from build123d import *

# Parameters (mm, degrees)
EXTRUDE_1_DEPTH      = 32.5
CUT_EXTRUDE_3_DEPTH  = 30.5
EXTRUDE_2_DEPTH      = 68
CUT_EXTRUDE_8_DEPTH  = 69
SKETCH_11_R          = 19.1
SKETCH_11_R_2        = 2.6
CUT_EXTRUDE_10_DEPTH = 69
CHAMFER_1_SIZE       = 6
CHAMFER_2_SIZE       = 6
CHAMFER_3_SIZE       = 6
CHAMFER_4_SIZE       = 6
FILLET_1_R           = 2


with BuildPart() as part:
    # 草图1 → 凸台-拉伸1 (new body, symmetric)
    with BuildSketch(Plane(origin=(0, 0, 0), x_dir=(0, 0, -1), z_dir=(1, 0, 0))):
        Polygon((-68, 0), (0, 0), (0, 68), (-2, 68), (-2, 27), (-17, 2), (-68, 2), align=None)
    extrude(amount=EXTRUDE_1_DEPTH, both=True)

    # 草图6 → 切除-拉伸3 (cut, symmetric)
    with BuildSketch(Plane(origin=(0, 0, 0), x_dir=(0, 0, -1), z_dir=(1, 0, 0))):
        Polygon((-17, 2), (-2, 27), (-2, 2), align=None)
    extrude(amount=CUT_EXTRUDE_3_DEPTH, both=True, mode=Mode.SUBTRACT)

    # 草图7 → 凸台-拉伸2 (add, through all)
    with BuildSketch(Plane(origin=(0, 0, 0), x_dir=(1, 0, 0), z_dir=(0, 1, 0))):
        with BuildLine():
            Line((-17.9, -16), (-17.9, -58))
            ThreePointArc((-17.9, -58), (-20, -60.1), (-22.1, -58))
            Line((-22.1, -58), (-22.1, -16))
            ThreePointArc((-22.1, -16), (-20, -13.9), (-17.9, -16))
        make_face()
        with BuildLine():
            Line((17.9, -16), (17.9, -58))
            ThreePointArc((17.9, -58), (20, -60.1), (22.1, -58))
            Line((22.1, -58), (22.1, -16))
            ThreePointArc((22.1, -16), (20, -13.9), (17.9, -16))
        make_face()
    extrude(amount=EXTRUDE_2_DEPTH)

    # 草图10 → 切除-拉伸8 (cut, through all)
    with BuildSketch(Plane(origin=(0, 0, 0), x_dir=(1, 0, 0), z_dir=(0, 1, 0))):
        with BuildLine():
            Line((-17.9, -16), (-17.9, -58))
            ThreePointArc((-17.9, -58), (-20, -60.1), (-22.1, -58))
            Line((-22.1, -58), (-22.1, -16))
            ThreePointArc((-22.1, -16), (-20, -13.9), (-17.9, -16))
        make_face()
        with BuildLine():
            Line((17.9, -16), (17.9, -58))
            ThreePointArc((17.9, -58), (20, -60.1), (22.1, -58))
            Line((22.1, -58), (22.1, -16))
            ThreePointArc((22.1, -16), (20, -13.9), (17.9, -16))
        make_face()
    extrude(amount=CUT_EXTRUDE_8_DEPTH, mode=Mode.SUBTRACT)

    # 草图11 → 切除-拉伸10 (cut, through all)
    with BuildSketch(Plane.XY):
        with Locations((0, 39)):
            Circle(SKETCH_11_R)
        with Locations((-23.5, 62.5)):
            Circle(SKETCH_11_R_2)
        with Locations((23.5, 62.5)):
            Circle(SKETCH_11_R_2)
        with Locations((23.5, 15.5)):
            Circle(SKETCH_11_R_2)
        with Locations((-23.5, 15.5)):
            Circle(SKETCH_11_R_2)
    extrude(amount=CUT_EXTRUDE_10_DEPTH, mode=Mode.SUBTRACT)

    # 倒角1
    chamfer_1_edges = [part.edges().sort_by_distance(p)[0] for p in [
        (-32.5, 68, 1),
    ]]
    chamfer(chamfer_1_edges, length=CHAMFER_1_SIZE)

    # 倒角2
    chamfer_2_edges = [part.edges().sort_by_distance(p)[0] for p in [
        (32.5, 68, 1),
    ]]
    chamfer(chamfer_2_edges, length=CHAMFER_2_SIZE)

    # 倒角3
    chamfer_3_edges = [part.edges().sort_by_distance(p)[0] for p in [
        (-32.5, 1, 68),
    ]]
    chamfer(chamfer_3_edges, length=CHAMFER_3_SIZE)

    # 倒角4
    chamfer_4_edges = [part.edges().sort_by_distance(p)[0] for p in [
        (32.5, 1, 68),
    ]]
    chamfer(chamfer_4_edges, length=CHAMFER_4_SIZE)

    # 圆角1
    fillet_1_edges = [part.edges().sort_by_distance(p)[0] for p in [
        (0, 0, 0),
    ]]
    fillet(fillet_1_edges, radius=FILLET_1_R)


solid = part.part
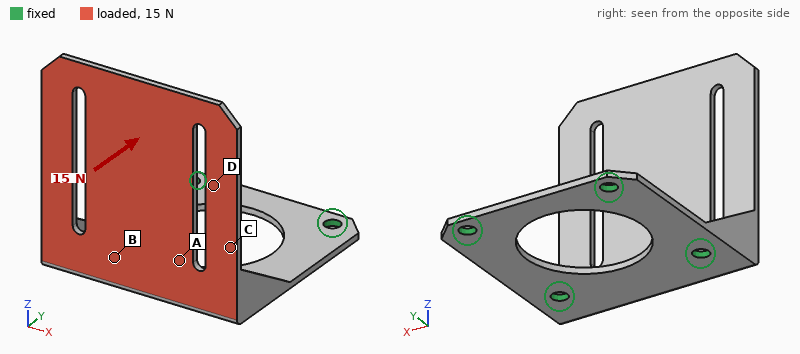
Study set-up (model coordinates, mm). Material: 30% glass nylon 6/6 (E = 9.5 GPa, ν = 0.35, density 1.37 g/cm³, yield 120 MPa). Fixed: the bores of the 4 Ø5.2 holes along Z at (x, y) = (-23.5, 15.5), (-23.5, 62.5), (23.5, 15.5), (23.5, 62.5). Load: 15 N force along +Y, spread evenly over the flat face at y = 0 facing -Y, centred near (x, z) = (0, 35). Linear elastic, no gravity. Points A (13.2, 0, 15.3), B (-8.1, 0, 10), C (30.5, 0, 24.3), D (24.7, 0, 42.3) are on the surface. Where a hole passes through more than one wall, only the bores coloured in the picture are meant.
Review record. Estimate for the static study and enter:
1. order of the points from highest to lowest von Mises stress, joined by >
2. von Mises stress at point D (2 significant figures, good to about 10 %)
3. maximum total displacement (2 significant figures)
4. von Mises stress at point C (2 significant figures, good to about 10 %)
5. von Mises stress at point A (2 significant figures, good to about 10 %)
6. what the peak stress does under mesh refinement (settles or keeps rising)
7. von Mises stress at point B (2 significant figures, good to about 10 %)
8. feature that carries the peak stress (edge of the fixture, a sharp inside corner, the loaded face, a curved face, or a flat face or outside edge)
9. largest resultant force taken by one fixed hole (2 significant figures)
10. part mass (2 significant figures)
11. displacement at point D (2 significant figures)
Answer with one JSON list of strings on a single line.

["C > A > B > D", "2.9 MPa", "1.4 mm", "8.6 MPa", "6.6 MPa", "keeps rising", "5.1 MPa", "a sharp inside corner", "9.1 N", "20 g", "0.60 mm"]
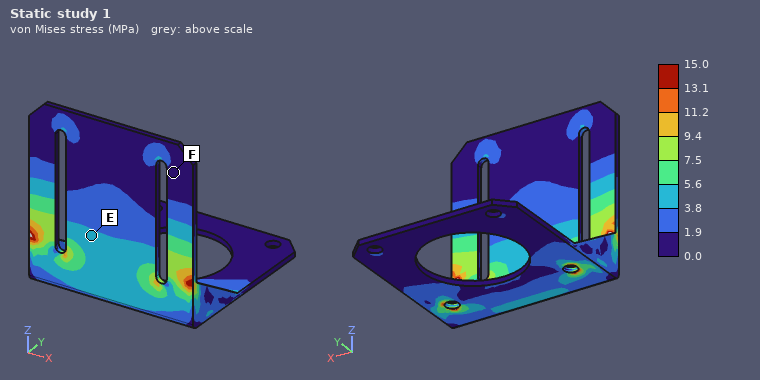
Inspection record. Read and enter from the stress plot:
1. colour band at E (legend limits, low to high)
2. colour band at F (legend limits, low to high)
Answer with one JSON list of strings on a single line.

["3.8 to 5.6 MPa", "0.0 to 1.9 MPa"]
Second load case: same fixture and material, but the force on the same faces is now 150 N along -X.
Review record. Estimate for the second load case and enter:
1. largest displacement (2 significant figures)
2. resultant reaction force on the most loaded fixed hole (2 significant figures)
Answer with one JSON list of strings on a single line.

["0.71 mm", "130 N"]
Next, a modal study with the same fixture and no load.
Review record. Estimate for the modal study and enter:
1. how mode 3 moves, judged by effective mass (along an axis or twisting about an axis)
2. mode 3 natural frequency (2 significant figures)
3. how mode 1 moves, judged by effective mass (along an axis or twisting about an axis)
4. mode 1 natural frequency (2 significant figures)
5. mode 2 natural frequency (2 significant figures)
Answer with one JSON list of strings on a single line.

["along X", "880 Hz", "along Y", "200 Hz", "530 Hz"]
